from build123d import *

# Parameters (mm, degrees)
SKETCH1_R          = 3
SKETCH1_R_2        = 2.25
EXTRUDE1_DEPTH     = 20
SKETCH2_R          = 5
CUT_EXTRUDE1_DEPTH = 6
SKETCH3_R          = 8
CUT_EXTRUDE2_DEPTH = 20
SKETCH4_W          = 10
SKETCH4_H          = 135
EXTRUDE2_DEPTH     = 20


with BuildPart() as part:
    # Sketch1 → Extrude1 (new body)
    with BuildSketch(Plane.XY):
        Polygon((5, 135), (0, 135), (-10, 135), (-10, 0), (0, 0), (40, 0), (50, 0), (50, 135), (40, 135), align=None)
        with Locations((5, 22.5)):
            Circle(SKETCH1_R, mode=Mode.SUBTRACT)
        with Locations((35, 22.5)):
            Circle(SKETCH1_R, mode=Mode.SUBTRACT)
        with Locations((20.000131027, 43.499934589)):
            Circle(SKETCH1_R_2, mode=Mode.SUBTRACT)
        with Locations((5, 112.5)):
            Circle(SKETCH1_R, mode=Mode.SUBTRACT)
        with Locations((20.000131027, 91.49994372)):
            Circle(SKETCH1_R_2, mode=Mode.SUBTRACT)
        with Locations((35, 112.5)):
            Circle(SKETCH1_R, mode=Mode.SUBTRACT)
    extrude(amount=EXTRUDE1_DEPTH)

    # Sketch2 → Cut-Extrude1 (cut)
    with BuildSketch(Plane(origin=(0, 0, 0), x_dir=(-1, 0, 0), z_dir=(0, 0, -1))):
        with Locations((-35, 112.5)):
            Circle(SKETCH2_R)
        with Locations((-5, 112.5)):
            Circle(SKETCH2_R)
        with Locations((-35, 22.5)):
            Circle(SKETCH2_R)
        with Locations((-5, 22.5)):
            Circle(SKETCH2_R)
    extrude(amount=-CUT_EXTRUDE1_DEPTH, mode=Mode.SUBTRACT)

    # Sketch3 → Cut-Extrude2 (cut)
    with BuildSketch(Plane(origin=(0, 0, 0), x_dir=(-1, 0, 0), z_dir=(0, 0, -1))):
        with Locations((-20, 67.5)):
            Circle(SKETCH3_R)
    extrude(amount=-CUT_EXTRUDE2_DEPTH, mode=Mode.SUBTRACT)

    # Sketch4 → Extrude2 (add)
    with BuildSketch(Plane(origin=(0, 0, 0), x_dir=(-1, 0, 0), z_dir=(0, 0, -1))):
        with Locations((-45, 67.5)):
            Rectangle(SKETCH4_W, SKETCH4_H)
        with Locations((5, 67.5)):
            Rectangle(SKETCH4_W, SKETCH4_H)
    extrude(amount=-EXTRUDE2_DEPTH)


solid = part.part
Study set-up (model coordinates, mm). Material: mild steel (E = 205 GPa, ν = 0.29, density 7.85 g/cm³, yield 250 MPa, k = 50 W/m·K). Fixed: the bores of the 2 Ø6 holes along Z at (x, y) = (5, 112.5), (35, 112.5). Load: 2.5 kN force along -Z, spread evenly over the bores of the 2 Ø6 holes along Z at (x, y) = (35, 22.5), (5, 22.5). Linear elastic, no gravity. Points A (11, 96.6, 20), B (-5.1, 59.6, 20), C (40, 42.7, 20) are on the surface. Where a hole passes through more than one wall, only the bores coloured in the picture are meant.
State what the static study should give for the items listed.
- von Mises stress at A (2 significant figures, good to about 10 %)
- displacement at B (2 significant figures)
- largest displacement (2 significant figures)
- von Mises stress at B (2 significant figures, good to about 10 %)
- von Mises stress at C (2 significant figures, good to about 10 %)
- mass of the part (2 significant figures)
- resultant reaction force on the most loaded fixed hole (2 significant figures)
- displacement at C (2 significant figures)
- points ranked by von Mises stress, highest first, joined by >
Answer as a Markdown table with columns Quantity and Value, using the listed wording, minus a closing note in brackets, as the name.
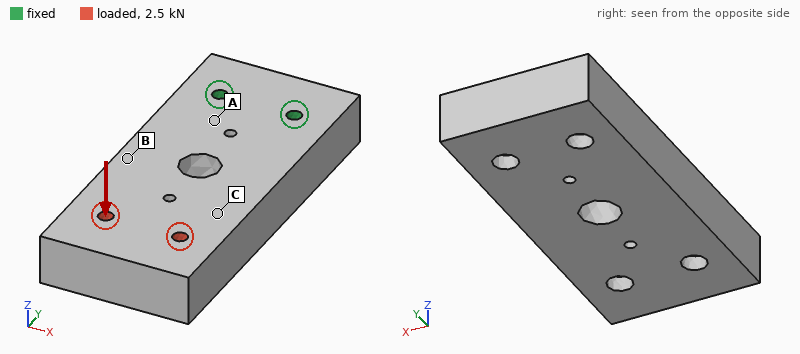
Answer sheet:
| Quantity | Value |
|---|---|
| von Mises stress at A | 47 MPa |
| displacement at B | 0.055 mm |
| largest displacement | 0.16 mm |
| von Mises stress at B | 28 MPa |
| von Mises stress at C | 14 MPa |
| mass of the part | 1.2 kg |
| resultant reaction force on the most loaded fixed hole | 1.3 kN |
| displacement at C | 0.083 mm |
| points ranked by von Mises stress, highest first, joined by > | A > B > C |
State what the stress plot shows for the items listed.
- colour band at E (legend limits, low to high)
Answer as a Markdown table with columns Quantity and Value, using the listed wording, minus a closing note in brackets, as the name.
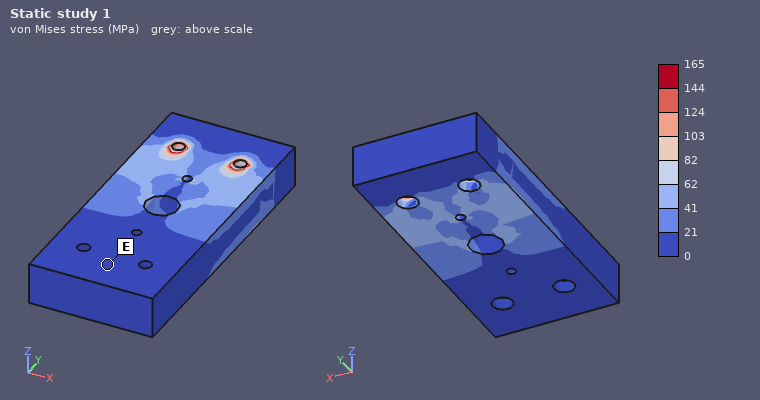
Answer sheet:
| Quantity | Value |
|---|---|
| colour band at E | 0 to 21 MPa |
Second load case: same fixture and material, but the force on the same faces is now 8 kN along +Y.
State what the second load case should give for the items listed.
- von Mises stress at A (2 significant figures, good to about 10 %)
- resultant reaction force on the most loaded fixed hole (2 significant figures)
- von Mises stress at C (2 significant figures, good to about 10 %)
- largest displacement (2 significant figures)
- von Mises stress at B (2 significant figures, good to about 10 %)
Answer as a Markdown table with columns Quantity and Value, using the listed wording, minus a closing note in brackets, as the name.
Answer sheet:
| Quantity | Value |
|---|---|
| von Mises stress at A | 13 MPa |
| resultant reaction force on the most loaded fixed hole | 4.0 kN |
| von Mises stress at C | 14 MPa |
| largest displacement | 19 µm |
| von Mises stress at B | 15 MPa |
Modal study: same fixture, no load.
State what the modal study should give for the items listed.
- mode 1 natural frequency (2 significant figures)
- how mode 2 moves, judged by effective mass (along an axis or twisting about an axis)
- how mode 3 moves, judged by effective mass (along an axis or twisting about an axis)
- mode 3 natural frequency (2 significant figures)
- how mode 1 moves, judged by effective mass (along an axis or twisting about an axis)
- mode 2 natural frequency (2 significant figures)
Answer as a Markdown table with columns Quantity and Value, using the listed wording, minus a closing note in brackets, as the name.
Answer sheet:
| Quantity | Value |
|---|---|
| mode 1 natural frequency | 1000 Hz |
| how mode 2 moves, judged by effective mass | along X |
| how mode 3 moves, judged by effective mass | twisting about Y |
| mode 3 natural frequency | 3900 Hz |
| how mode 1 moves, judged by effective mass | along Z |
| mode 2 natural frequency | 2700 Hz |
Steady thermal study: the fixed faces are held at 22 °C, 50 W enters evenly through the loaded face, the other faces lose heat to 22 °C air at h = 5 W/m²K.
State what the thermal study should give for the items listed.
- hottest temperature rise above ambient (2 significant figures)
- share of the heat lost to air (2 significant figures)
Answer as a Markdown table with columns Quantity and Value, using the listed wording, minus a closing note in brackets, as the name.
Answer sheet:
| Quantity | Value |
|---|---|
| hottest temperature rise above ambient | 86 K |
| share of the heat lost to air | 10 % |
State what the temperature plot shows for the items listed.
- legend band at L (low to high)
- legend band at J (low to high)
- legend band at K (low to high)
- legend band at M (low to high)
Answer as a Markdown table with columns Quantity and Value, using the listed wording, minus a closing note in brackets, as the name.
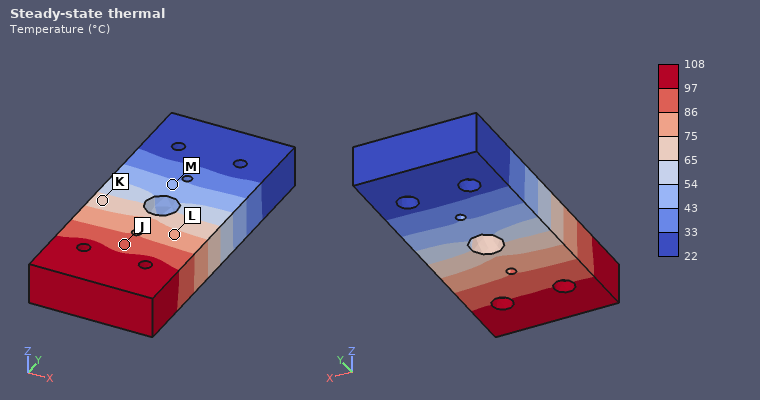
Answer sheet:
| Quantity | Value |
|---|---|
| legend band at L | 75 to 86 °C |
| legend band at J | 86 to 97 °C |
| legend band at K | 65 to 75 °C |
| legend band at M | 43 to 54 °C |
